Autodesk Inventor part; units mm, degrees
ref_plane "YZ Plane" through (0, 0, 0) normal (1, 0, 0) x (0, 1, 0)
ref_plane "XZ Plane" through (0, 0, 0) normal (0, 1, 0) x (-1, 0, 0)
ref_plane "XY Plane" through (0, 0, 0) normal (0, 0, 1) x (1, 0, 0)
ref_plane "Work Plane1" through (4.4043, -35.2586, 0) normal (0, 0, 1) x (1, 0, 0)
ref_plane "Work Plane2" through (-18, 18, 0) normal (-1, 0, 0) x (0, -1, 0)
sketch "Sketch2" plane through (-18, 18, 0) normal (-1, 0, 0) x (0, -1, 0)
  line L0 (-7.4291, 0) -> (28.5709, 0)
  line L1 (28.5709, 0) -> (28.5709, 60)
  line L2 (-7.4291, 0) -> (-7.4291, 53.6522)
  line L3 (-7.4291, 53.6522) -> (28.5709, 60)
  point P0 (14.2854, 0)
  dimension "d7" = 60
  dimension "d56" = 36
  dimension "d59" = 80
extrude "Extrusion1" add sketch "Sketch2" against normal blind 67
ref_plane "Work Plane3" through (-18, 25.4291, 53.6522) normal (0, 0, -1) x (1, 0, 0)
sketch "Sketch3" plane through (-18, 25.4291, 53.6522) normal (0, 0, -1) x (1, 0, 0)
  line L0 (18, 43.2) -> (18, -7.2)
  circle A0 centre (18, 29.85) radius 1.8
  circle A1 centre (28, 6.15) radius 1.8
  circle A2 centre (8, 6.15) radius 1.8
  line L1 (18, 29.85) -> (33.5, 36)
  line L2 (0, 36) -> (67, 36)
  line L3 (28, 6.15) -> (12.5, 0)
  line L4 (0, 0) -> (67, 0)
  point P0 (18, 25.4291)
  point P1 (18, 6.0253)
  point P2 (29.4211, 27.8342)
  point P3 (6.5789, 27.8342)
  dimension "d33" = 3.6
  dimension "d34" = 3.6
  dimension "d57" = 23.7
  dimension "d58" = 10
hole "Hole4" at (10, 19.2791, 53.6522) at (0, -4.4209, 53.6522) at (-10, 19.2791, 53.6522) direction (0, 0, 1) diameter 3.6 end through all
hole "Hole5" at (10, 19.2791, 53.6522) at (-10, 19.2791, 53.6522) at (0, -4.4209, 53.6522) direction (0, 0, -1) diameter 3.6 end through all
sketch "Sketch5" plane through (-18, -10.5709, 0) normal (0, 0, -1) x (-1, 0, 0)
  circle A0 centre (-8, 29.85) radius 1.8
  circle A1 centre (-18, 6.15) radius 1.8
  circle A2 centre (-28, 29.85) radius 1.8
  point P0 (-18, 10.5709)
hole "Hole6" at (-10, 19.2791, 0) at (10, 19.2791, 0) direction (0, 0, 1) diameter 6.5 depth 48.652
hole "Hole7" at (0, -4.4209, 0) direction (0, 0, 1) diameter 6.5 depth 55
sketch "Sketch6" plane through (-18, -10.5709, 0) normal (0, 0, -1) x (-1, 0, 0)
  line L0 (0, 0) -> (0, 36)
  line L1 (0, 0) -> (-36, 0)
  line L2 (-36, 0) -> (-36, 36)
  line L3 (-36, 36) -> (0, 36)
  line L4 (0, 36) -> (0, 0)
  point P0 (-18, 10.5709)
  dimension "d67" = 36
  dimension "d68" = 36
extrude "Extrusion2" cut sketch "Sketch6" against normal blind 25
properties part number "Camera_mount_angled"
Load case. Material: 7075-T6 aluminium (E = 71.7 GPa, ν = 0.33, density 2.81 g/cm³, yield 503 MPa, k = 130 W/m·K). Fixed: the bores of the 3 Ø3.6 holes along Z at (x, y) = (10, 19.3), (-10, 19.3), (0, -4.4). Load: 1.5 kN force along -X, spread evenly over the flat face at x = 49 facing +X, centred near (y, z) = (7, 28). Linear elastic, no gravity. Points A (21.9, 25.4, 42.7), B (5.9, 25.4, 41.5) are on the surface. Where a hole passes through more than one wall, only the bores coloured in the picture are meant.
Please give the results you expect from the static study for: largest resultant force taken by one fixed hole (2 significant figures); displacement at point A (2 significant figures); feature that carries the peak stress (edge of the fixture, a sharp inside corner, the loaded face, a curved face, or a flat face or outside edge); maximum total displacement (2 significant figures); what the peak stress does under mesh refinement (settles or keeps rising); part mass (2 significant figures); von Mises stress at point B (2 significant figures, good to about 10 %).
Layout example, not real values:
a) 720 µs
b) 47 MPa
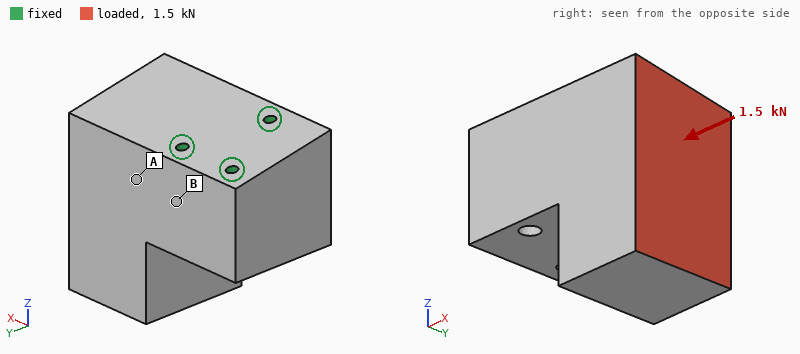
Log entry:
a) 1.7 kN
b) 7.5 µm
c) edge of the fixture
d) 31 µm
e) keeps rising
f) 290 g
g) 9.2 MPa
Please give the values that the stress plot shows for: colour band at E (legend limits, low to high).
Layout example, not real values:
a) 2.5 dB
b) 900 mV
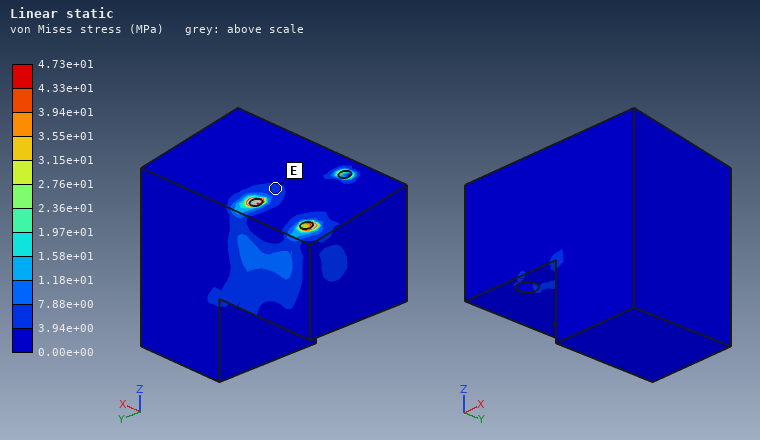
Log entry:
a) 3.94e+00 to 7.88e+00 MPa
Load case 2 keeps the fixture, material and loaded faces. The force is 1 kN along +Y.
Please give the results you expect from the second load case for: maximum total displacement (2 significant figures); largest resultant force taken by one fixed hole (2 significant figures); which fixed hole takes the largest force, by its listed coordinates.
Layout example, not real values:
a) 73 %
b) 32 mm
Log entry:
a) 22 µm
b) 1.8 kN
c) (10, 19.3)
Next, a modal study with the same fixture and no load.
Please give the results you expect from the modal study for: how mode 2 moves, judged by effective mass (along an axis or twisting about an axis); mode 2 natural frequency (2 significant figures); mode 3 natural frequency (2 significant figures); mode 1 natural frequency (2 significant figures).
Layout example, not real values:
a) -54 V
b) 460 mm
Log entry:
a) along Y
b) 3400 Hz
c) 7100 Hz
d) 2500 Hz
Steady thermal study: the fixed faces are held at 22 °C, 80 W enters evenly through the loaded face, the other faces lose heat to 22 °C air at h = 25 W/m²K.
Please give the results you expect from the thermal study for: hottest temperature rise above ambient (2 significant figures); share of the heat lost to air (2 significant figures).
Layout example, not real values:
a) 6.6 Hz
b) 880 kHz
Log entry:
a) 32 K
b) 7.6 %
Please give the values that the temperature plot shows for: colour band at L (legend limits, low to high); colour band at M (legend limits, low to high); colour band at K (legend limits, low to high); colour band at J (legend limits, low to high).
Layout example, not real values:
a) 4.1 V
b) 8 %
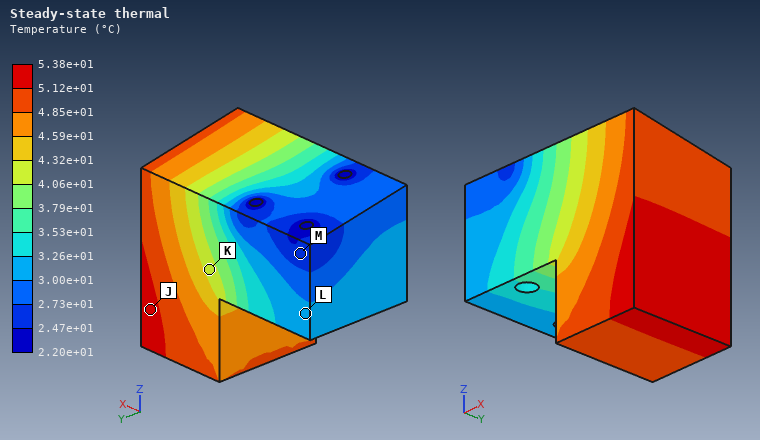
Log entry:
a) 3.00e+01 to 3.26e+01 °C
b) 2.47e+01 to 2.73e+01 °C
c) 4.06e+01 to 4.32e+01 °C
d) 5.12e+01 to 5.38e+01 °C
